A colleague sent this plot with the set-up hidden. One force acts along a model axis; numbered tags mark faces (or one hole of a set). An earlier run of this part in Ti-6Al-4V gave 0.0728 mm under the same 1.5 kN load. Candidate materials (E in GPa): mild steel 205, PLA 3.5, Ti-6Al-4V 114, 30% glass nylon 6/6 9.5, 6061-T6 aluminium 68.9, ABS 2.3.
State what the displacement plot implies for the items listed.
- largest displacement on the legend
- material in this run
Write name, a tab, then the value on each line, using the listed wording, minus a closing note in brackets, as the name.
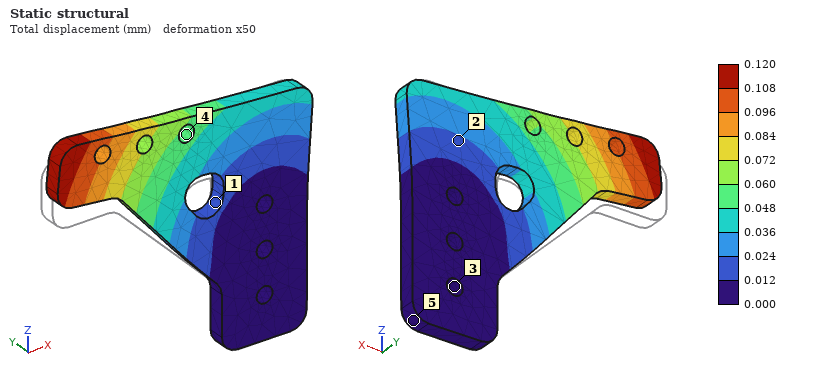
largest displacement on the legend	0.120 mm
material in this run	6061-T6 aluminium
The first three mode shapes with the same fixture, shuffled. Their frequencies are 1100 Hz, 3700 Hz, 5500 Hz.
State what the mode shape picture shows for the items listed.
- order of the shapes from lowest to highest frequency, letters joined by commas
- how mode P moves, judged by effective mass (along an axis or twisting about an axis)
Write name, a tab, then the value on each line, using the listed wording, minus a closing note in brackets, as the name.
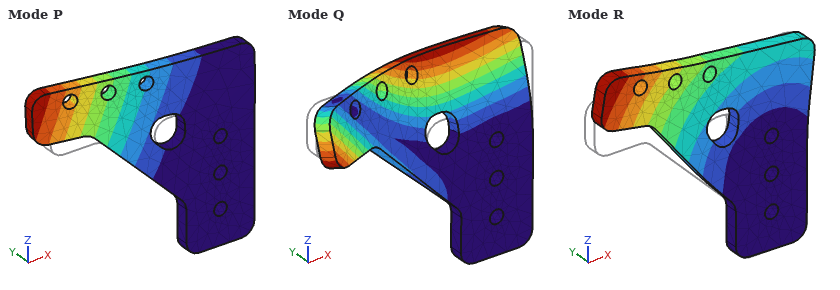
order of the shapes from lowest to highest frequency, letters joined by commas	P, Q, R
how mode P moves, judged by effective mass	along Y
